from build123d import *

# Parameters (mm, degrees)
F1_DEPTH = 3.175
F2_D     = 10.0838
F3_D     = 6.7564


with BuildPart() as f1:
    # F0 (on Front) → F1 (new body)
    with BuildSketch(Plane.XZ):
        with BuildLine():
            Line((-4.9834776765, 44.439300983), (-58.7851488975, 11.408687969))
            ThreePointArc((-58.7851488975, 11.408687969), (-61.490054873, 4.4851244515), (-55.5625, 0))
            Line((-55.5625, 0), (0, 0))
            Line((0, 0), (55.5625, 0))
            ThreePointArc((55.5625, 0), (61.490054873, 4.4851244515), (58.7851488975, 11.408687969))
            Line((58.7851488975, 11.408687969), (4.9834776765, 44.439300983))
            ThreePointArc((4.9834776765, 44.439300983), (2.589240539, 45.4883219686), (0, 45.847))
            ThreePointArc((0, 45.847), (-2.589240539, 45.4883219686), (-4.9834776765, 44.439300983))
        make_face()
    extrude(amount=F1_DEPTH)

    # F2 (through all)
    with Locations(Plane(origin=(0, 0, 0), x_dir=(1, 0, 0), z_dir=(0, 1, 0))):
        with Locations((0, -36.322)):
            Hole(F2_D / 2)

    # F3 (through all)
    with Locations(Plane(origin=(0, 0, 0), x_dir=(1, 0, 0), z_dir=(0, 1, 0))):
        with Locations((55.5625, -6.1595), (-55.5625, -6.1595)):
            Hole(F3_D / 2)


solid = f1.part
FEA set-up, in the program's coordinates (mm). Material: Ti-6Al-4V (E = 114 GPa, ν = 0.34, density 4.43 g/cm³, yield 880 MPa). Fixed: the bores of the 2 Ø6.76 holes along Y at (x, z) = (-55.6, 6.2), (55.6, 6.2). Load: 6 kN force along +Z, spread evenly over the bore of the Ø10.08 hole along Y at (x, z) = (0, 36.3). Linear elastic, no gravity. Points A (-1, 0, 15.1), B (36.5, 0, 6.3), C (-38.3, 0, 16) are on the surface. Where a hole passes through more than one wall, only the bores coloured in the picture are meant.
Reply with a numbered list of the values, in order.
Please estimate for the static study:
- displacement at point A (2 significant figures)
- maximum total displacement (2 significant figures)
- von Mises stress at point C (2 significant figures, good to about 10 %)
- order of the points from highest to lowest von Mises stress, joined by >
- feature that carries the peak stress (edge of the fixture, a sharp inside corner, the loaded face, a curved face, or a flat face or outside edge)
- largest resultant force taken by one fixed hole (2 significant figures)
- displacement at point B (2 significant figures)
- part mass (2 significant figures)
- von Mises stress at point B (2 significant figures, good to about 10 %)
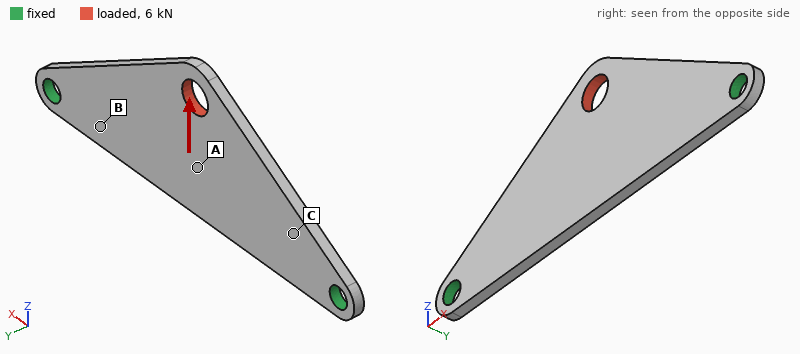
1. 0.097 mm
2. 0.10 mm
3. 92 MPa
4. C > B > A
5. edge of the fixture
6. 4.4 kN
7. 0.048 mm
8. 47 g
9. 57 MPa
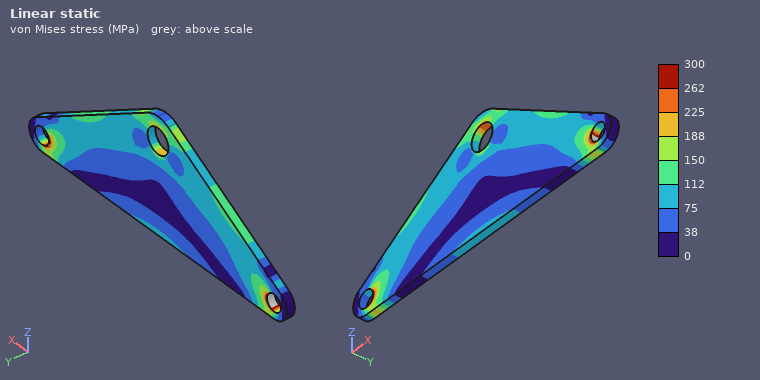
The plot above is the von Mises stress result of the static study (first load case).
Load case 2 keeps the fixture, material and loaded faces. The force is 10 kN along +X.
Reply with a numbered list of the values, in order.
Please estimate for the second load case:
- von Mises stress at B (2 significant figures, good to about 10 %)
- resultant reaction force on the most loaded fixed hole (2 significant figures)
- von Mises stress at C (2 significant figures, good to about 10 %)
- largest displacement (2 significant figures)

1. 54 MPa
2. 5.7 kN
3. 110 MPa
4. 89 µm
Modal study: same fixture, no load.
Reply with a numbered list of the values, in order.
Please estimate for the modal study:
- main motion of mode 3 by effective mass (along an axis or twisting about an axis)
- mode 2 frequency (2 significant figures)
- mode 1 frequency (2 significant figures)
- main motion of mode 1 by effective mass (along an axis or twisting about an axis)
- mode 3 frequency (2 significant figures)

1. twisting about Z
2. 2100 Hz
3. 970 Hz
4. along Y
5. 3200 Hz
